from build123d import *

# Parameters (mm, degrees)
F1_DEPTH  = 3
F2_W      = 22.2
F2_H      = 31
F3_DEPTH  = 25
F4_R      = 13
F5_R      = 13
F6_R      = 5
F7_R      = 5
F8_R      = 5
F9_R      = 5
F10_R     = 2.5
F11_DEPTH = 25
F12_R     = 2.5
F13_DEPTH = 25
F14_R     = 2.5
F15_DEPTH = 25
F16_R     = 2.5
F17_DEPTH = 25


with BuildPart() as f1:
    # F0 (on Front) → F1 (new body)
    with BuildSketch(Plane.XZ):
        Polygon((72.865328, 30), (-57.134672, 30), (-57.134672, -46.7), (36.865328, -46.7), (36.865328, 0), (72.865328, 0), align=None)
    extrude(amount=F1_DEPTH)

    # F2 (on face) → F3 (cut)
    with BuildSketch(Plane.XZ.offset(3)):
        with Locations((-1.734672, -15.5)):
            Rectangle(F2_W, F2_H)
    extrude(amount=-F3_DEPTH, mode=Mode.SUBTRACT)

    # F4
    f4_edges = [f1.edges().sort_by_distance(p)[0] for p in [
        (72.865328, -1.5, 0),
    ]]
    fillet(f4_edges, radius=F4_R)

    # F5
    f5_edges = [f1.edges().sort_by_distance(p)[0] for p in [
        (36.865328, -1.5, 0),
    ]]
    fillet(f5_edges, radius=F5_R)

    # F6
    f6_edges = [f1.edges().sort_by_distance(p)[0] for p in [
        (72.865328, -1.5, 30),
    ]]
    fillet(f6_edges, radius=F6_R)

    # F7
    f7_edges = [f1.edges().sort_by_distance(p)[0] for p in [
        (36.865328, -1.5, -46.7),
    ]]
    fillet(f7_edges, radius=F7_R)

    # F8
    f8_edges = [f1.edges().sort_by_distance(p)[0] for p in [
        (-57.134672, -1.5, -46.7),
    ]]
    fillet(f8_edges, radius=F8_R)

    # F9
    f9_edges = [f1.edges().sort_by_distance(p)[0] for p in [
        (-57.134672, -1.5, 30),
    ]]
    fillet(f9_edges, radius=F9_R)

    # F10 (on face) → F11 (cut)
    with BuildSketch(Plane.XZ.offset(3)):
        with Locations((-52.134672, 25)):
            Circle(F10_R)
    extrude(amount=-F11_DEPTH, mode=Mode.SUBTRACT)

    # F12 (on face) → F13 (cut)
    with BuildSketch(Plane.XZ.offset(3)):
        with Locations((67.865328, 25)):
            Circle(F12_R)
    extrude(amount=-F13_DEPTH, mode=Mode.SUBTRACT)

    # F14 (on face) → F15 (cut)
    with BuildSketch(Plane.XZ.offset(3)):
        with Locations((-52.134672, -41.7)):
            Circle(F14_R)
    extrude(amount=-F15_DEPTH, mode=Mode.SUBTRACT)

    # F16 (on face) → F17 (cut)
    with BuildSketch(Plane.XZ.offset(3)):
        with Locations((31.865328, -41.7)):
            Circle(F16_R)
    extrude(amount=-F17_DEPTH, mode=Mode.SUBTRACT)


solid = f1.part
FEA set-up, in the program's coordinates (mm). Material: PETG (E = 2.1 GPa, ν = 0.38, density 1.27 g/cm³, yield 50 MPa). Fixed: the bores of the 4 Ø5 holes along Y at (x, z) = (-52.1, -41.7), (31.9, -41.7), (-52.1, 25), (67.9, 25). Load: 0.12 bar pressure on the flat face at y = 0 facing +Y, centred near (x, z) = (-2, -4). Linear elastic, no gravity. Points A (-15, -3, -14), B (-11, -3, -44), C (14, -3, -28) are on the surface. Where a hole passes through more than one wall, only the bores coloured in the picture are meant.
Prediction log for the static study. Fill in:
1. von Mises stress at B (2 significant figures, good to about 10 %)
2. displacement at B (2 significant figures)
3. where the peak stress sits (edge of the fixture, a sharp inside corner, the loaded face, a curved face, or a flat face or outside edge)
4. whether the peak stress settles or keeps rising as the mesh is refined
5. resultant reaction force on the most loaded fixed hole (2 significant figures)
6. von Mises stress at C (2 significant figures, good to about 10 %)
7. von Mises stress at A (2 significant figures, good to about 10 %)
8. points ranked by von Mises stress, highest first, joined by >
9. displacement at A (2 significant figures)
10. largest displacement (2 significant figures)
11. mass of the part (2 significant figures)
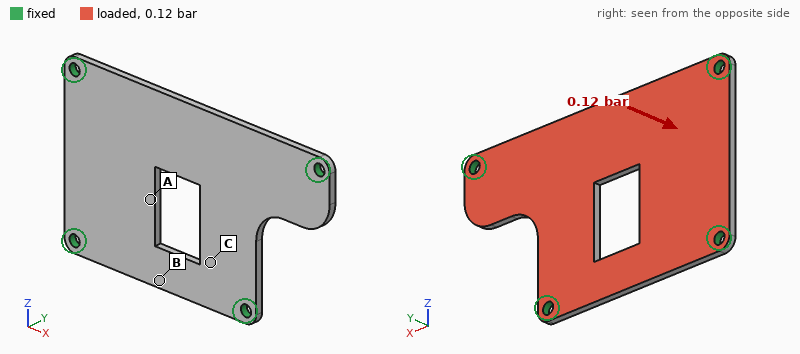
3.9 MPa
0.45 mm
edge of the fixture
keeps rising
27 N
1.2 MPa
2.4 MPa
B > A > C
0.94 mm
1.5 mm
29 g
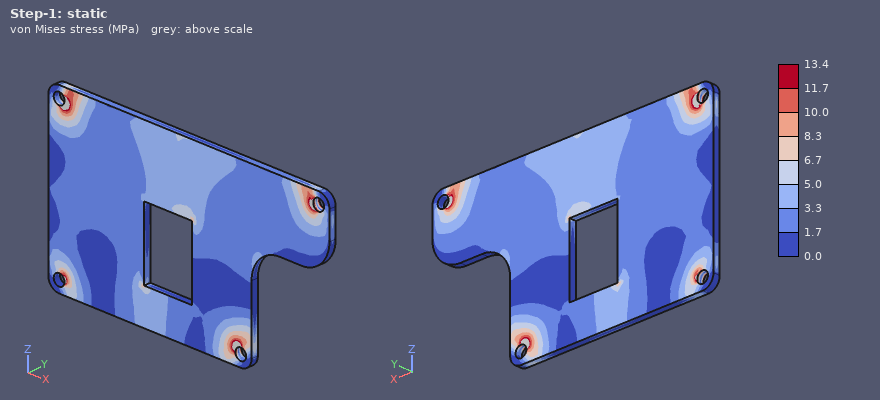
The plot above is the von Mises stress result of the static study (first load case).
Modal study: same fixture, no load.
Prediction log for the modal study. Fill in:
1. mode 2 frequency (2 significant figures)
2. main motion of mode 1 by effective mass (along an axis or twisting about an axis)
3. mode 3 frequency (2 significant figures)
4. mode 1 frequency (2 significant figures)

560 Hz
along Y
730 Hz
300 Hz
